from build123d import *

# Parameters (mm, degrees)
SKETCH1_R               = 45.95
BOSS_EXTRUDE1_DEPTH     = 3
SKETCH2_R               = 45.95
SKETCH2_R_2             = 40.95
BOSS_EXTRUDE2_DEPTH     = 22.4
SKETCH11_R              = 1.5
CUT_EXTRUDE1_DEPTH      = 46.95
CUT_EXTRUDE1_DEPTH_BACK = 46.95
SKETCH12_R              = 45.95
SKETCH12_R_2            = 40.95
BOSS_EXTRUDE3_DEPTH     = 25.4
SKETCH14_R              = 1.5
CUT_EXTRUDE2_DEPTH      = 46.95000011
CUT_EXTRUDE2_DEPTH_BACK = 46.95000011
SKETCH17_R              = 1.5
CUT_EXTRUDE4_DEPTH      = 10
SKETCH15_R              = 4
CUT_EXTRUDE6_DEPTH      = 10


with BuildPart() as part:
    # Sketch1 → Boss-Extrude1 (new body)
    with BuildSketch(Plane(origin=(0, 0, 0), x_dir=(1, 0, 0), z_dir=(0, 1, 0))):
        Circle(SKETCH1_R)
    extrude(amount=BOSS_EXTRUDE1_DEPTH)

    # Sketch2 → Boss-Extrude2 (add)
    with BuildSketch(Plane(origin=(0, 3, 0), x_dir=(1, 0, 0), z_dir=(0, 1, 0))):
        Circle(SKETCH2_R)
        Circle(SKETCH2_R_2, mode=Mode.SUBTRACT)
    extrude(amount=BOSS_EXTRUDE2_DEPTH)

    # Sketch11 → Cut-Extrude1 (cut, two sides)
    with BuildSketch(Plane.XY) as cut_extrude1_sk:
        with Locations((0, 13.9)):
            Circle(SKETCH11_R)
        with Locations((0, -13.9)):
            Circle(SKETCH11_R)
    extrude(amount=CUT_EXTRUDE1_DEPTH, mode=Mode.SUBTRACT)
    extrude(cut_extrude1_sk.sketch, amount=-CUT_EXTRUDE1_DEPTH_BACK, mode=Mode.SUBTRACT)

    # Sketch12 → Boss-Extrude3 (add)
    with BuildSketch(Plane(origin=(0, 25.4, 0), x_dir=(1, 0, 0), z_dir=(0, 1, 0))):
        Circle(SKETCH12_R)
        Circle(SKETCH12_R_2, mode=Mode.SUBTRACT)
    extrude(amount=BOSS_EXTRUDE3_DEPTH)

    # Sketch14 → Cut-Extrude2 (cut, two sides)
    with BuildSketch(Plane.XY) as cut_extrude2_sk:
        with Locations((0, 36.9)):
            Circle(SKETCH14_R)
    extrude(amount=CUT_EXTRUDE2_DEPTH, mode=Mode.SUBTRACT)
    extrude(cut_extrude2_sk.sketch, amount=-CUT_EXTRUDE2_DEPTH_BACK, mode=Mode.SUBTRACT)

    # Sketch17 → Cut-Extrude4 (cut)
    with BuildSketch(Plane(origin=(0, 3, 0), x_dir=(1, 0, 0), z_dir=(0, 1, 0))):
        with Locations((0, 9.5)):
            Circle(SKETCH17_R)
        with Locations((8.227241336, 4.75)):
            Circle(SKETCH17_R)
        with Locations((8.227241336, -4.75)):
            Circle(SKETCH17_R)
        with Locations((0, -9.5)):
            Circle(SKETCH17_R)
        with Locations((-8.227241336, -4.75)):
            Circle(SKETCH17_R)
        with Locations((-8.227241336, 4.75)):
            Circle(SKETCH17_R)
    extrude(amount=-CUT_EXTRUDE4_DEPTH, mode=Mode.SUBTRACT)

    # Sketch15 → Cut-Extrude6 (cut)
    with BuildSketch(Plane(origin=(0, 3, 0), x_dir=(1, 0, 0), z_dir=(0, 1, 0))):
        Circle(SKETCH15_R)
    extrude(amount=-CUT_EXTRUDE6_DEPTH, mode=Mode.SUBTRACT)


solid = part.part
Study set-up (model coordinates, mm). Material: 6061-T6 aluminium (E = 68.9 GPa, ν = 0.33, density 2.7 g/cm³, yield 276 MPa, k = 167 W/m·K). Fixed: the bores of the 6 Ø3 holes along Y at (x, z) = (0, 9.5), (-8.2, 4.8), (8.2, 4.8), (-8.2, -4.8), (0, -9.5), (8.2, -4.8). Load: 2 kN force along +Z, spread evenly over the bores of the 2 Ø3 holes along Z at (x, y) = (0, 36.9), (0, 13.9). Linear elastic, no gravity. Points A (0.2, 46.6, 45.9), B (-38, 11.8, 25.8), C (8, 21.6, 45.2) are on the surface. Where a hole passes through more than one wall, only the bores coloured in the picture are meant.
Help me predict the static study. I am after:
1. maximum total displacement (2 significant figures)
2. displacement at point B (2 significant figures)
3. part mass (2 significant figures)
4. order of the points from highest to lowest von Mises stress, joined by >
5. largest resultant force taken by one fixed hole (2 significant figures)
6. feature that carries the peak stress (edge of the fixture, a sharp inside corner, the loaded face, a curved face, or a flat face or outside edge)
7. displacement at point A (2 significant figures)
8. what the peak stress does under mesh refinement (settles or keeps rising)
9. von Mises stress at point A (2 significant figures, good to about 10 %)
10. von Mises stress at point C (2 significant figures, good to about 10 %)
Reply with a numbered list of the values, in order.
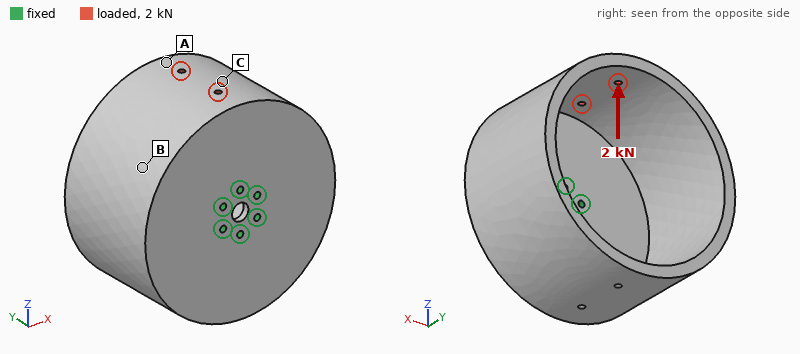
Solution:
1. 1.1 mm
2. 0.37 mm
3. 230 g
4. A > C > B
5. 920 N
6. edge of the fixture
7. 1.0 mm
8. keeps rising
9. 62 MPa
10. 33 MPa
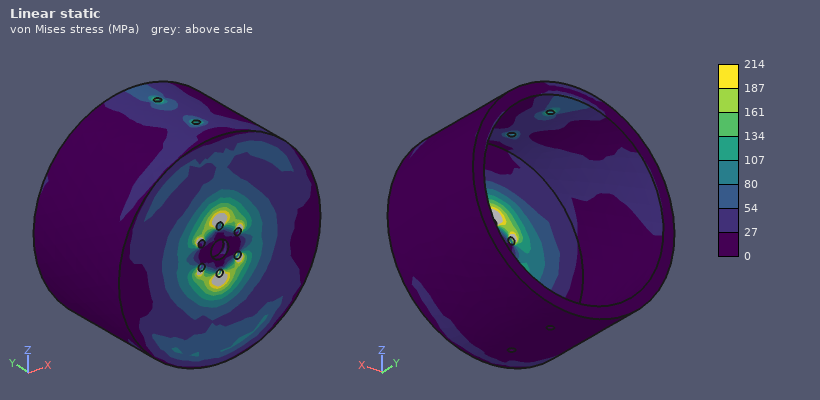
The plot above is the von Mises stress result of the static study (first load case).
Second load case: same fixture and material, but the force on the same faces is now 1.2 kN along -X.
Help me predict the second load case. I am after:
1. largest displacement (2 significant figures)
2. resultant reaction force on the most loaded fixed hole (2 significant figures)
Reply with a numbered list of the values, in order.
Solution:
1. 0.56 mm
2. 1.2 kN
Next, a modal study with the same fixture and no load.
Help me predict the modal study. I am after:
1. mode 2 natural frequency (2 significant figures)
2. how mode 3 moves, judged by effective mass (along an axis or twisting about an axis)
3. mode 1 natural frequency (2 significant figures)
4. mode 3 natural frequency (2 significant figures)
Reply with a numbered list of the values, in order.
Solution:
1. 520 Hz
2. along Y
3. 510 Hz
4. 1100 Hz
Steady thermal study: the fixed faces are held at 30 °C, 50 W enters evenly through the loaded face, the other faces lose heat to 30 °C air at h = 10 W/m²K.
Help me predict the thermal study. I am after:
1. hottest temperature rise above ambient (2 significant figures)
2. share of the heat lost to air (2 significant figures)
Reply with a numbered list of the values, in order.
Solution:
1. 51 K
2. 16 %
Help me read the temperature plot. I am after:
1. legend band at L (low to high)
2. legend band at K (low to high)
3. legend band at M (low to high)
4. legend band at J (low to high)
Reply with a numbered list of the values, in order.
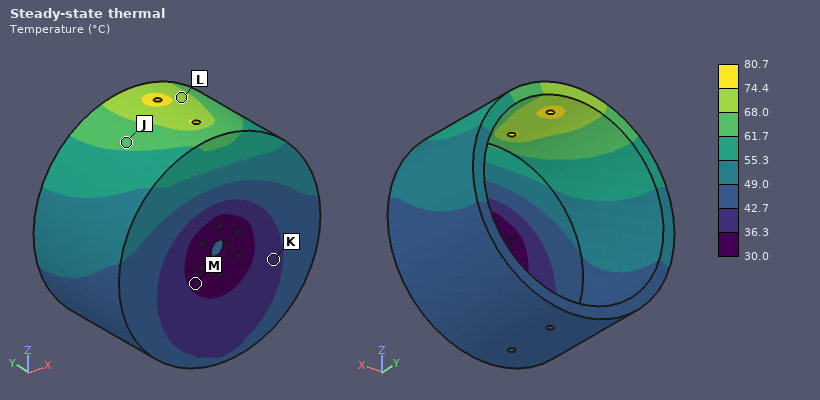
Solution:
1. 68.0 to 74.4 °C
2. 36.3 to 42.7 °C
3. 30.0 to 36.3 °C
4. 61.7 to 68.0 °C
